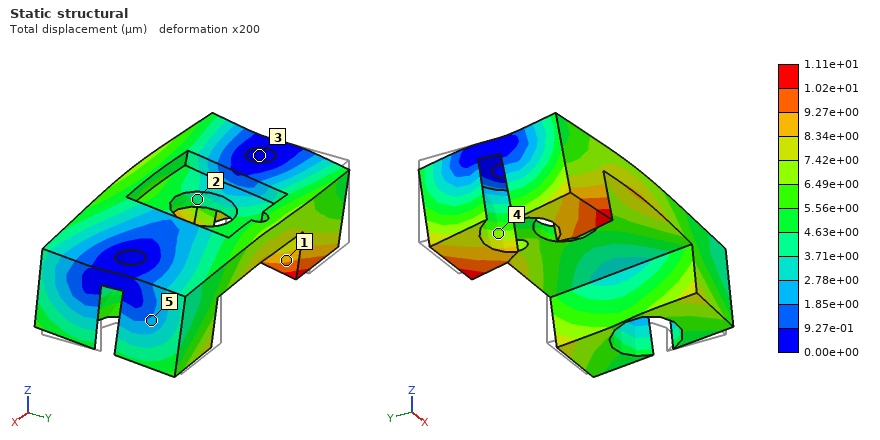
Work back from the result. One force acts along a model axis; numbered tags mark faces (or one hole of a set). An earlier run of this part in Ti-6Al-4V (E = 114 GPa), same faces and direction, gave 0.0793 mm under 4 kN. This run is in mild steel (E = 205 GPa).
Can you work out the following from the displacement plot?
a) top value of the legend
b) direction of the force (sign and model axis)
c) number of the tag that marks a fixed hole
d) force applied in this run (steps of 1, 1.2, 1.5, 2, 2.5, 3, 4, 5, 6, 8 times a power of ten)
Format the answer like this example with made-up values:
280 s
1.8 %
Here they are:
1.11e+01 µm
-Y
3
1 kN
